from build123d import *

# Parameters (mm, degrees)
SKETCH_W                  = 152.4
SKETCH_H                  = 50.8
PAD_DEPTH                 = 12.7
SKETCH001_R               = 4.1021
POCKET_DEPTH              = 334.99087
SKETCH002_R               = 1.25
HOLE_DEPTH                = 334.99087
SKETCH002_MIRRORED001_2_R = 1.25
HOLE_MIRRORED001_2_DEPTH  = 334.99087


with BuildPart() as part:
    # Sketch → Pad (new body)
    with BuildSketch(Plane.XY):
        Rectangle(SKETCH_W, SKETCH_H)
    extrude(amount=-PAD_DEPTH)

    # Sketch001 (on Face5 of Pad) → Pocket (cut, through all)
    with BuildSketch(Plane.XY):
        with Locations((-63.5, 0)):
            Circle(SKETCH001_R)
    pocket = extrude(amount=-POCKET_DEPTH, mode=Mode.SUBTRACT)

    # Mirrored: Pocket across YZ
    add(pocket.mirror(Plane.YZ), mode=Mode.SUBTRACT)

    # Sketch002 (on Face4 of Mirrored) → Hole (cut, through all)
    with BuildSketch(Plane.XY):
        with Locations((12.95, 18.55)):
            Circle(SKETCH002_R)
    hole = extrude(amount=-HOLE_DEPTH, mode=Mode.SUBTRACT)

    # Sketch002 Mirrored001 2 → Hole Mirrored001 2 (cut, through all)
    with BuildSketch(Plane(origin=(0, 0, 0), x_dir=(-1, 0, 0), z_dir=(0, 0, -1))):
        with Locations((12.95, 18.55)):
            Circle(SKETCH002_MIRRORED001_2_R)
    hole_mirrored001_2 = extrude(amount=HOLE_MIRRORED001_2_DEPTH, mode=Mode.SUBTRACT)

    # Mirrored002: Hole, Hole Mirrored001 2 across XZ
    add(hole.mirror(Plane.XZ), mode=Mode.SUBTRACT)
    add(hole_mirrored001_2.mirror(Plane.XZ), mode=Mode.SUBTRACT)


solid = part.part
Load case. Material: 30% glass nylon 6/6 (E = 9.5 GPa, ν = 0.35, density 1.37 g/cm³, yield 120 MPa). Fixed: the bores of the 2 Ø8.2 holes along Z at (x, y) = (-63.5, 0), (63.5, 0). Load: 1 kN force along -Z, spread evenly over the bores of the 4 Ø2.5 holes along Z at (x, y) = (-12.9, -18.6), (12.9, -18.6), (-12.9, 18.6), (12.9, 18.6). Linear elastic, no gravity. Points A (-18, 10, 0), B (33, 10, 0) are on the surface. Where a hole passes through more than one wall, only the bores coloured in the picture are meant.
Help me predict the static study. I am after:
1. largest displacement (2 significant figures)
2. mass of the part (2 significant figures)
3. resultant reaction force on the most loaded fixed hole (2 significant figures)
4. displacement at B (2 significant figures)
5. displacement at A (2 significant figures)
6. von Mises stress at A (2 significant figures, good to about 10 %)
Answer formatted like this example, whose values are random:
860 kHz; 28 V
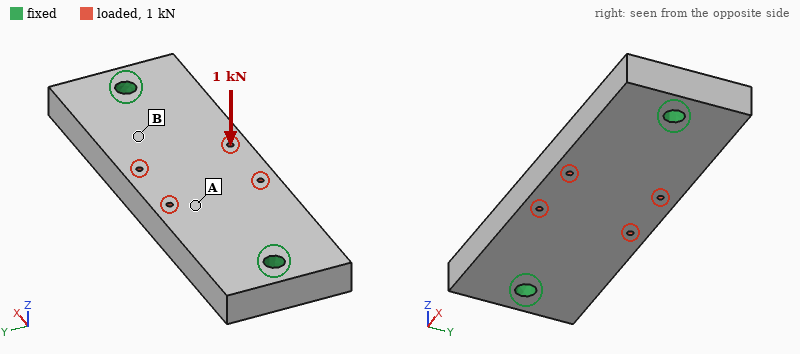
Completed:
0.16 mm; 130 g; 500 N; 0.082 mm; 0.12 mm; 6.4 MPa
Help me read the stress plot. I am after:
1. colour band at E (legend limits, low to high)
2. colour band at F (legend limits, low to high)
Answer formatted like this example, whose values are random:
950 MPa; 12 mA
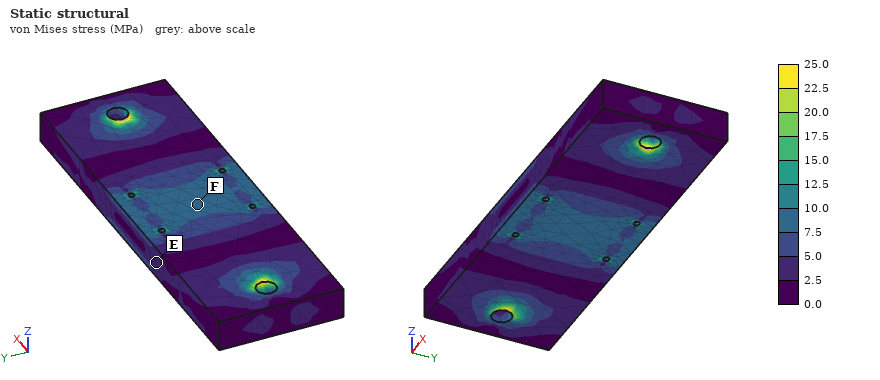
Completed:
2.5 to 5.0 MPa; 7.5 to 10.0 MPa
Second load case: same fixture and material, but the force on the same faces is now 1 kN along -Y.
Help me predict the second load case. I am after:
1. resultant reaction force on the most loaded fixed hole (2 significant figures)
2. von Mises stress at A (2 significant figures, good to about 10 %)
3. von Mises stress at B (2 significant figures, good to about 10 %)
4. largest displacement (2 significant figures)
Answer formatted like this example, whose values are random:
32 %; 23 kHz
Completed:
500 N; 2.0 MPa; 1.9 MPa; 36 µm
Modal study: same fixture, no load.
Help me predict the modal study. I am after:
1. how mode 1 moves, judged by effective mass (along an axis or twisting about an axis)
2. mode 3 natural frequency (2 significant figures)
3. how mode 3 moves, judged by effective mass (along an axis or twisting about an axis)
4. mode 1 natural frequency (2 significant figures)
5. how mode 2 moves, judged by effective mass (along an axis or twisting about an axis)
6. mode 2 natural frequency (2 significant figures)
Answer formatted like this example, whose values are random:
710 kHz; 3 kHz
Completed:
along Z; 3400 Hz; along Y; 1800 Hz; twisting about X; 2700 Hz
